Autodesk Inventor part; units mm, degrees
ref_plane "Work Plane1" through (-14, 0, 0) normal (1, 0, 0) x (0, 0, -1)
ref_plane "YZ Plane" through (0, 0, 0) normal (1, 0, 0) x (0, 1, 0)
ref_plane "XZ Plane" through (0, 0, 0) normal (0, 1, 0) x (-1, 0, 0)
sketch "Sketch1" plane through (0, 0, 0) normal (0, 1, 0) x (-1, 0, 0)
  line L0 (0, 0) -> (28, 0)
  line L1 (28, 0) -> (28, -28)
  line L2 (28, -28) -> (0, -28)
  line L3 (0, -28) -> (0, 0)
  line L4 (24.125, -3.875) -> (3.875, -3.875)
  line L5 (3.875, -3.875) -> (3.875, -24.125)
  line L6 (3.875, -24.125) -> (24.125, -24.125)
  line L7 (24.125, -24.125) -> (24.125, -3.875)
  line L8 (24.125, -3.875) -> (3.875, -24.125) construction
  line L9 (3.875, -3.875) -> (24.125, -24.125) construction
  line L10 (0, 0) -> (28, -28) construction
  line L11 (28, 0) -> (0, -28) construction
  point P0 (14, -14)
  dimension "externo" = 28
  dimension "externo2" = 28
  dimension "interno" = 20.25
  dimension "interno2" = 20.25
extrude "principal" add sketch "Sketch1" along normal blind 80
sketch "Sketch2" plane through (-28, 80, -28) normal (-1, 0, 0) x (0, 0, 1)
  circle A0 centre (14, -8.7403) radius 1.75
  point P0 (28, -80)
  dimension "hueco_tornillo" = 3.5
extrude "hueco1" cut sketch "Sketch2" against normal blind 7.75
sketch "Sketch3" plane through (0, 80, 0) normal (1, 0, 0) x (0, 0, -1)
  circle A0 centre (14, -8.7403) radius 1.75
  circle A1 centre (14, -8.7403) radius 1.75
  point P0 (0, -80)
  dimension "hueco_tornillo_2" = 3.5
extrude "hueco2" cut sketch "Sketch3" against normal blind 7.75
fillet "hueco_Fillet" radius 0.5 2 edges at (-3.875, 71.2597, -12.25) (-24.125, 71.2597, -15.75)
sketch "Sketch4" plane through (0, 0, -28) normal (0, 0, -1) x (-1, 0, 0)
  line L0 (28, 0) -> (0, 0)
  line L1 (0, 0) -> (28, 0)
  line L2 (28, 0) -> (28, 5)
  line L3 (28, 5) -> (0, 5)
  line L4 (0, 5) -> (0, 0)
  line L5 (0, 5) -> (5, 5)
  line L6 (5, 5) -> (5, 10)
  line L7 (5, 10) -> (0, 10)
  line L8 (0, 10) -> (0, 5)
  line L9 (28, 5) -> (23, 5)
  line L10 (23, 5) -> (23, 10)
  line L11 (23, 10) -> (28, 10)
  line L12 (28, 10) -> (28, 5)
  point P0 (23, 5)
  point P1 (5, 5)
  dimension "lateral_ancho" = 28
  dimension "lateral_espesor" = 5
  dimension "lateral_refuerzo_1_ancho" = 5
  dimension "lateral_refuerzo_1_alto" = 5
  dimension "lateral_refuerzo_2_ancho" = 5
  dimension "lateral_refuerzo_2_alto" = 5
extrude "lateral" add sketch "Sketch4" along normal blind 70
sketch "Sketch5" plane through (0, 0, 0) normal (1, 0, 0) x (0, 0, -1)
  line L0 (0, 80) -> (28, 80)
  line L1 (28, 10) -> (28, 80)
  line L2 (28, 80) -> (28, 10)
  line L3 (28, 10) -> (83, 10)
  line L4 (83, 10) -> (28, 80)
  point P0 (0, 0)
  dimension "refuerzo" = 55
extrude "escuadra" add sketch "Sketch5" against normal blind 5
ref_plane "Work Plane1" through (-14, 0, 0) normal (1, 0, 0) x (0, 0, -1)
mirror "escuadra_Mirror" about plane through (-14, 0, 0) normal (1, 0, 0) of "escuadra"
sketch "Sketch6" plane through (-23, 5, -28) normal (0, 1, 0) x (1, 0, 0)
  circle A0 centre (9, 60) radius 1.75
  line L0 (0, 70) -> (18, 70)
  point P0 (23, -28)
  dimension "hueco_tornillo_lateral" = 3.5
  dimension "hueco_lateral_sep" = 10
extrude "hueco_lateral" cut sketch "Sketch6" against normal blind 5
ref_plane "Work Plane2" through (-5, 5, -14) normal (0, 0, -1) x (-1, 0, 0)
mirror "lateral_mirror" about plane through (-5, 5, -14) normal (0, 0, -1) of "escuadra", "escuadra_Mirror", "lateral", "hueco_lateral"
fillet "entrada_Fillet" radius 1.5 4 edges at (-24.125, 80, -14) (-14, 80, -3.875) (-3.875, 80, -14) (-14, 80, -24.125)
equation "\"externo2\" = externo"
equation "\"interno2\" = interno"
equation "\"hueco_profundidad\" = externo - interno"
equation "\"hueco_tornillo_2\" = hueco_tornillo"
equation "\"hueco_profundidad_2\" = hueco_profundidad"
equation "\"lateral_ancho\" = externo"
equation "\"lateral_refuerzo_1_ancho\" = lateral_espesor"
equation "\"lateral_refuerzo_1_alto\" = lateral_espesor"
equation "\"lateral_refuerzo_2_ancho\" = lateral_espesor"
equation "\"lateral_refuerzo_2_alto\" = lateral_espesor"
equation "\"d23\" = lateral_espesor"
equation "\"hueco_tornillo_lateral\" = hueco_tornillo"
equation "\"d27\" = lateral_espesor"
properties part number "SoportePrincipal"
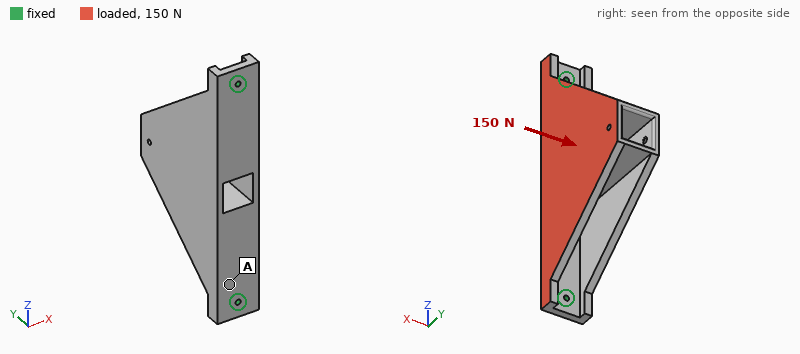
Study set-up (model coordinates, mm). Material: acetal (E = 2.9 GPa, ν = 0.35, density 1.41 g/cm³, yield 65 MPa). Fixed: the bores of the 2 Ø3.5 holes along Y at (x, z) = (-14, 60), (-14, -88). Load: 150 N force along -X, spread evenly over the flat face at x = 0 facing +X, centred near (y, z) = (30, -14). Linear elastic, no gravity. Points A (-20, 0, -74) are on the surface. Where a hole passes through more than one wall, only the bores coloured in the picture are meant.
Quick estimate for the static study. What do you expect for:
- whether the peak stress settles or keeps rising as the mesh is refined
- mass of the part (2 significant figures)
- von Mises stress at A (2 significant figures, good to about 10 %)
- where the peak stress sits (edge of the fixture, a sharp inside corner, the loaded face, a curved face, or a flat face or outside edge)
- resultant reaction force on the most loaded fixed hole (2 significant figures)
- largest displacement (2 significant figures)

keeps rising
130 g
2.4 MPa
edge of the fixture
75 N
1.9 mm
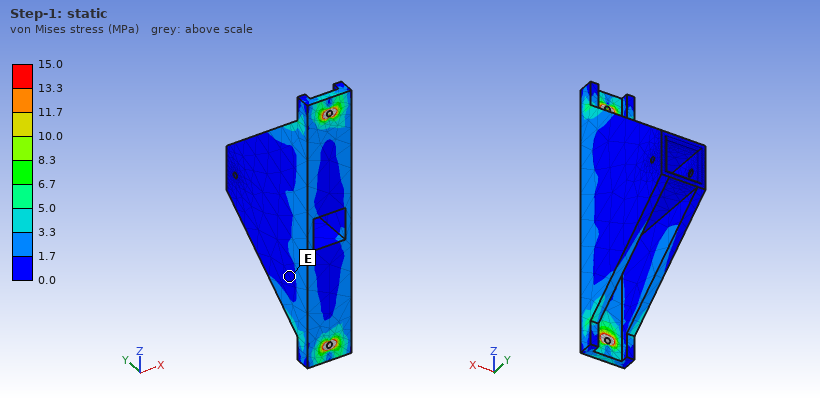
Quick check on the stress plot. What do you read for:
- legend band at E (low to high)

0.0 to 1.7 MPa
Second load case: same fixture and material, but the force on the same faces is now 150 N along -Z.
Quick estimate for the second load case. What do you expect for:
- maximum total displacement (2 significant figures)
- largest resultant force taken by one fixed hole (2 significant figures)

30 µm
81 N
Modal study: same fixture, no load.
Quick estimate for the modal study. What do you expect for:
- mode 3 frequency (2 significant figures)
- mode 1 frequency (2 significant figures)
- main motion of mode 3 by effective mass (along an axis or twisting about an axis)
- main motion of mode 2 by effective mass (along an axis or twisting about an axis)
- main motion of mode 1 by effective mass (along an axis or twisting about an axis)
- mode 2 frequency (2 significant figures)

990 Hz
170 Hz
along X
along Y
along X
810 Hz
